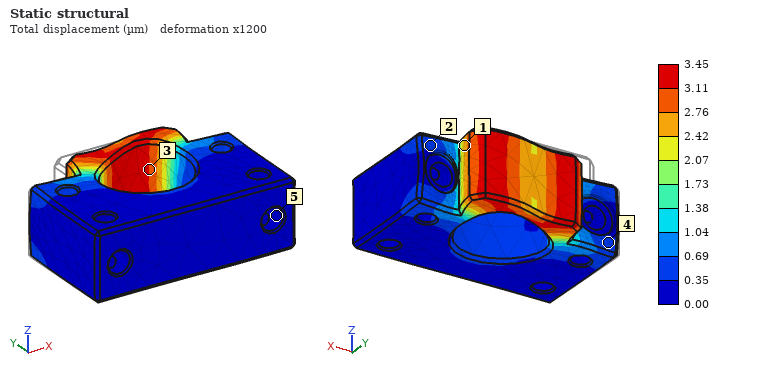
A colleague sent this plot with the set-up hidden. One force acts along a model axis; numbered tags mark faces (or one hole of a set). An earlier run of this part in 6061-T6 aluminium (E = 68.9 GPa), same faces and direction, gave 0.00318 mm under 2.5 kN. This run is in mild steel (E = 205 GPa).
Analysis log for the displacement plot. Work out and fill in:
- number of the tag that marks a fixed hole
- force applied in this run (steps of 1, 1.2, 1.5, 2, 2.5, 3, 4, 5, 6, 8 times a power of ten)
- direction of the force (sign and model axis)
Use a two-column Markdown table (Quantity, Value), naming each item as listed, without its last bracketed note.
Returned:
| Quantity | Value |
|---|---|
| number of the tag that marks a fixed hole | 5 |
| force applied in this run | 8 kN |
| direction of the force | +X |
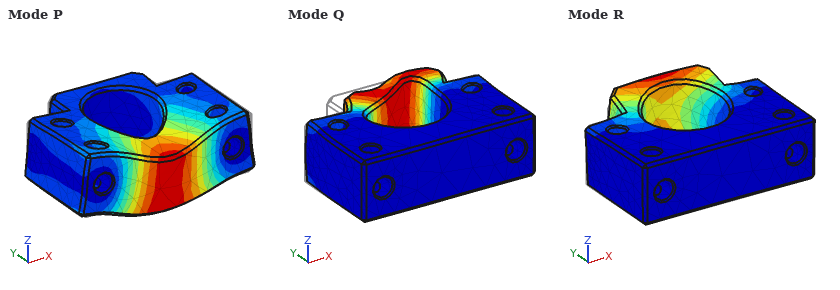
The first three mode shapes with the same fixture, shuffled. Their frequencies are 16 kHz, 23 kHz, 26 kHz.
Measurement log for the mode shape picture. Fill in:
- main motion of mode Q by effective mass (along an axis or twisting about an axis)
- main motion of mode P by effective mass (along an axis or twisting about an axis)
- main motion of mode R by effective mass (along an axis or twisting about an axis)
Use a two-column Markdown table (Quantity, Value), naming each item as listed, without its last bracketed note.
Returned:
| Quantity | Value |
|---|---|
| main motion of mode Q by effective mass | along X |
| main motion of mode P by effective mass | along Z |
| main motion of mode R by effective mass | along Z |
